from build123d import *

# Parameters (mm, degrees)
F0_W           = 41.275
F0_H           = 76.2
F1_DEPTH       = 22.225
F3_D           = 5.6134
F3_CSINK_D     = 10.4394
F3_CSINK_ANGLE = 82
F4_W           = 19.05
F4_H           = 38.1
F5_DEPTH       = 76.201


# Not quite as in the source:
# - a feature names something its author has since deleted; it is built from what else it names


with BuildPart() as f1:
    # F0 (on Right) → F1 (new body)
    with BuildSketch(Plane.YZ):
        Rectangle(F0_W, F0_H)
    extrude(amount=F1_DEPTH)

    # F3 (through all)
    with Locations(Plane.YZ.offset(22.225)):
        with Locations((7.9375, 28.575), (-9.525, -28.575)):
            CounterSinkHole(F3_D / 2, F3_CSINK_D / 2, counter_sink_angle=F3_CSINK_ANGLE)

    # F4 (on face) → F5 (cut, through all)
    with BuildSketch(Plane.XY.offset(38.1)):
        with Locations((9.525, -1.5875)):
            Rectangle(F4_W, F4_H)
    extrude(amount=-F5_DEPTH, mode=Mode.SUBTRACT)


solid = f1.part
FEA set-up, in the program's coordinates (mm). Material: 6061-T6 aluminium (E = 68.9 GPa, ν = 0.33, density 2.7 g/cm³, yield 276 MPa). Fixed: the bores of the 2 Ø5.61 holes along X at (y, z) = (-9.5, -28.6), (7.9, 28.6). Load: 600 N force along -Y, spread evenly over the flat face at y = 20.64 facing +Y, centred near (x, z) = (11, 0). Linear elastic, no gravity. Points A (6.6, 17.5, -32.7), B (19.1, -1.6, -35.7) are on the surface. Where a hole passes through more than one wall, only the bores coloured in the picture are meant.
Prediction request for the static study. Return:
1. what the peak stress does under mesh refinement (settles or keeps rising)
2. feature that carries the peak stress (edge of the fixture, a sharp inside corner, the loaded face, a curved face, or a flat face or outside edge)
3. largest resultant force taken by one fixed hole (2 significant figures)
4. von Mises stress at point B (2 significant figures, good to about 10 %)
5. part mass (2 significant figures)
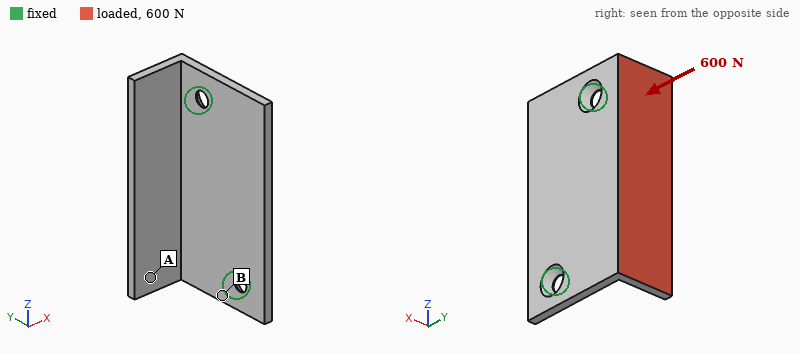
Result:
keeps rising
edge of the fixture
320 N
48 MPa
39 g
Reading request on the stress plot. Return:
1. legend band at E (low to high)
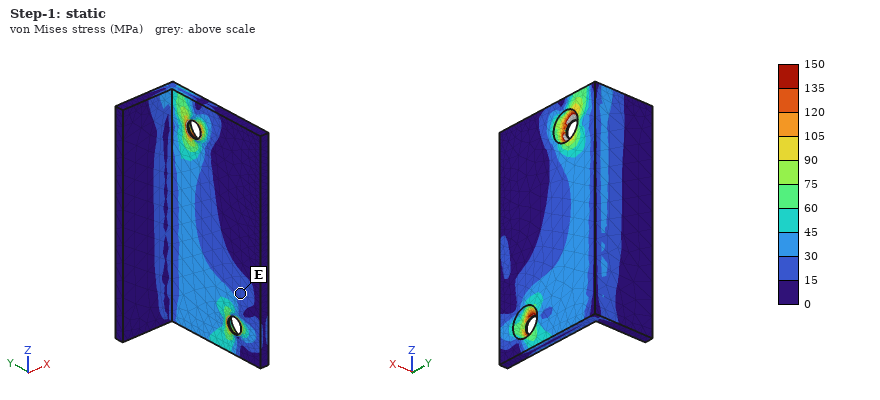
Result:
15 to 30 MPa
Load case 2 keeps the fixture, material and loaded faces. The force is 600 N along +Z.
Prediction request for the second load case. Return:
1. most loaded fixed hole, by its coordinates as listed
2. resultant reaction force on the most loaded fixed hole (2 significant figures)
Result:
(7.9, 28.6)
580 N
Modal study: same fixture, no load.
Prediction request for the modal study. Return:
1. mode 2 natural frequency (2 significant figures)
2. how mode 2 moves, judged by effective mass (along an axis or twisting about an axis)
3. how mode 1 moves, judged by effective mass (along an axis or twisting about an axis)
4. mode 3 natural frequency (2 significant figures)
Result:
2400 Hz
along X
along X
3500 Hz
